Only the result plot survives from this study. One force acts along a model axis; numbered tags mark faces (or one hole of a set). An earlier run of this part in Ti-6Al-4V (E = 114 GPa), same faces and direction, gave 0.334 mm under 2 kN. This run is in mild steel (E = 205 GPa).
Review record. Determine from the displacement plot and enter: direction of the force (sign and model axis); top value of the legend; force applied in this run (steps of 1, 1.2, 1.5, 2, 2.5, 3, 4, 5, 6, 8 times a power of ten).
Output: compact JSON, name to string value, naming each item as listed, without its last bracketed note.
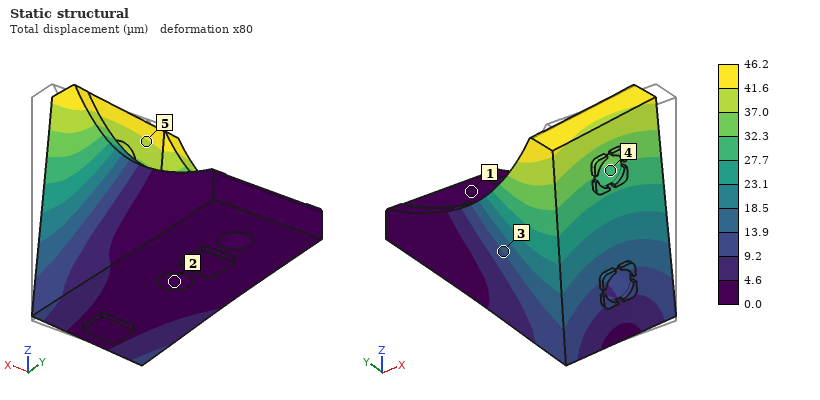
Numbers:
{"direction of the force": "-X", "top value of the legend": "46.2 µm", "force applied in this run": "500 N"}
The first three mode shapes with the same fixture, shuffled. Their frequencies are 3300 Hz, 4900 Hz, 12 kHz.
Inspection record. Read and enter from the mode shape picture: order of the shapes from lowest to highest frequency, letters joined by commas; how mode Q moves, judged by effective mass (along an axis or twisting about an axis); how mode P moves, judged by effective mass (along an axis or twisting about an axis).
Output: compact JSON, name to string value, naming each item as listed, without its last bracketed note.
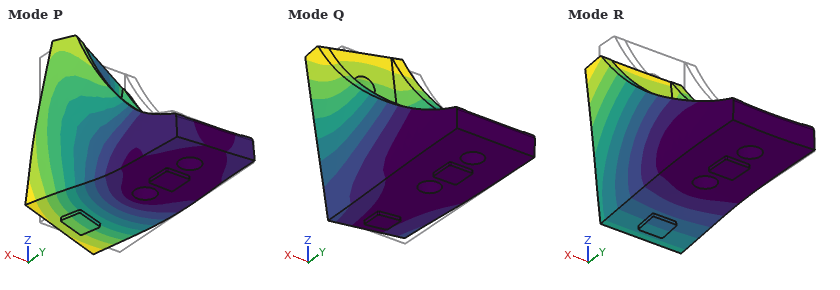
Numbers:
{"order of the shapes from lowest to highest frequency, letters joined by commas": "Q, R, P", "how mode Q moves, judged by effective mass": "along X", "how mode P moves, judged by effective mass": "along X"}
